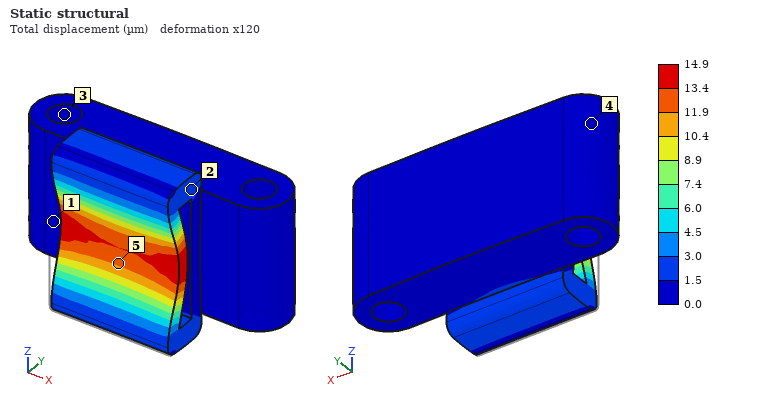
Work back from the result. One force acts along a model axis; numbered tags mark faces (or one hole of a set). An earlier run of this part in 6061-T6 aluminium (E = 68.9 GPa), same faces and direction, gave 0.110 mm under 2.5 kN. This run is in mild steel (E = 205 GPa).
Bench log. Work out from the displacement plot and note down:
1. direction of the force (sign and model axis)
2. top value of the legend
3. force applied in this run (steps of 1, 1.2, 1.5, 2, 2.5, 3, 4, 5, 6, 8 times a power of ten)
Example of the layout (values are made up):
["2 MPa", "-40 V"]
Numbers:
["+Y", "14.9 µm", "1 kN"]
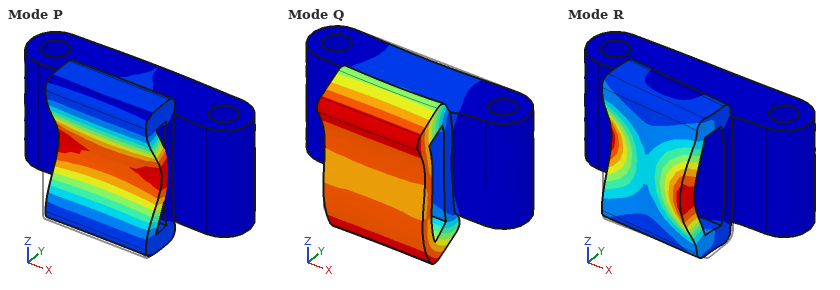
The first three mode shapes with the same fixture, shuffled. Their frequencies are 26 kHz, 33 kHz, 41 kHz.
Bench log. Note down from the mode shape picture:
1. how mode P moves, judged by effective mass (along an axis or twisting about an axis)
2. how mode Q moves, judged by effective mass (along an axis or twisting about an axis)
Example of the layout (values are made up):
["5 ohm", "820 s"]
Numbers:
["along Y", "along Z"]
